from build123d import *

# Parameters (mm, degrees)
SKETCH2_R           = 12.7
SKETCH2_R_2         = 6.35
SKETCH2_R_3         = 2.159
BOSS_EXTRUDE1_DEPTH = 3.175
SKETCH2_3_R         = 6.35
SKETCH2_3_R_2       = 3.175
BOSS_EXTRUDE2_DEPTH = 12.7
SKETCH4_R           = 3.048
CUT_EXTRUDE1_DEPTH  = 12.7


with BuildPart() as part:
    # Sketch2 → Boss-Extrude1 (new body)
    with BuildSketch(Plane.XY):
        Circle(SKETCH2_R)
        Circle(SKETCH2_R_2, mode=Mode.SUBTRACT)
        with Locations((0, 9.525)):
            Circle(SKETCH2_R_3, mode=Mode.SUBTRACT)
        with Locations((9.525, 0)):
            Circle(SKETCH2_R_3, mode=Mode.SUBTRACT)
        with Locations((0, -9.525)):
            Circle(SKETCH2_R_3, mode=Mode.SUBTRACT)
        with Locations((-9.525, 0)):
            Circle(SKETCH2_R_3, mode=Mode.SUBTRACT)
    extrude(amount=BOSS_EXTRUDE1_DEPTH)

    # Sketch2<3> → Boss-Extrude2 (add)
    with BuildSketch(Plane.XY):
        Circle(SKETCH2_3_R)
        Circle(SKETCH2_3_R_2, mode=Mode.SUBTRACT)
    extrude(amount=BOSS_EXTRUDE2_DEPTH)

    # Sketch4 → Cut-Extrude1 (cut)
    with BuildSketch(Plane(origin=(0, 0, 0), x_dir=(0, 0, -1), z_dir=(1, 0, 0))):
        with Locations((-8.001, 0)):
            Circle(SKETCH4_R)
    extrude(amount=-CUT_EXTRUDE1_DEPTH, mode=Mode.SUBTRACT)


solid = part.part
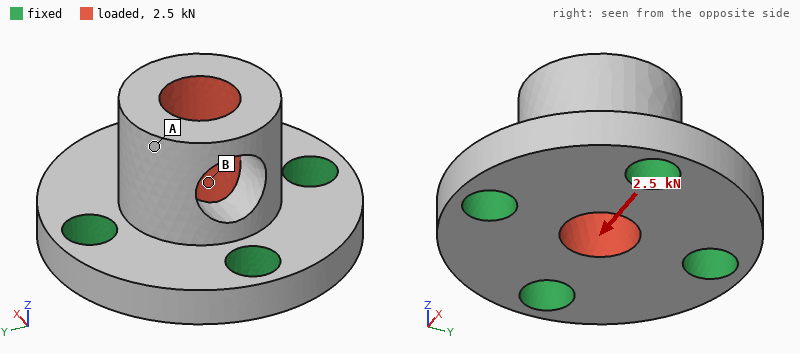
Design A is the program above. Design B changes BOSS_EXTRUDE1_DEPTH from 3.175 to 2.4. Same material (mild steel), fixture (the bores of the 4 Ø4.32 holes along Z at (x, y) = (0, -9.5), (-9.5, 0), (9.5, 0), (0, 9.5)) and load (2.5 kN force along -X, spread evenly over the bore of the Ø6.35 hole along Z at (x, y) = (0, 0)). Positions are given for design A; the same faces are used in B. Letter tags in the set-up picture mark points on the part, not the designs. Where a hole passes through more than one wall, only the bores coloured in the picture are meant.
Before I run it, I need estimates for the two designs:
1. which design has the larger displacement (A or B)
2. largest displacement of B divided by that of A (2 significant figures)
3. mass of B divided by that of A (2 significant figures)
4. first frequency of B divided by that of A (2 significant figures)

B
1.3
0.88
0.88
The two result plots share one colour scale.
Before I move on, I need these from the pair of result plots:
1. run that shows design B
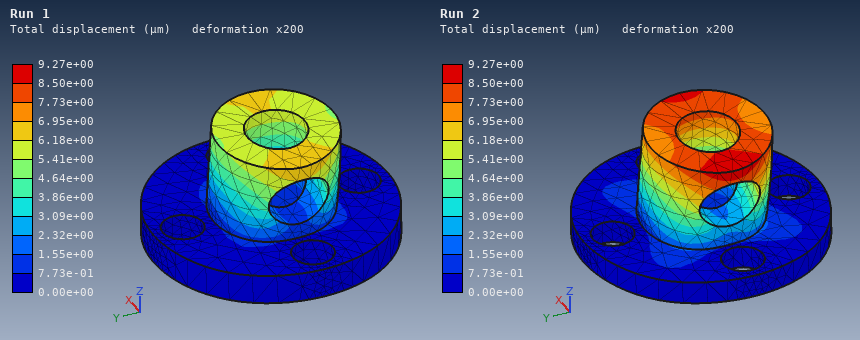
Run 2
